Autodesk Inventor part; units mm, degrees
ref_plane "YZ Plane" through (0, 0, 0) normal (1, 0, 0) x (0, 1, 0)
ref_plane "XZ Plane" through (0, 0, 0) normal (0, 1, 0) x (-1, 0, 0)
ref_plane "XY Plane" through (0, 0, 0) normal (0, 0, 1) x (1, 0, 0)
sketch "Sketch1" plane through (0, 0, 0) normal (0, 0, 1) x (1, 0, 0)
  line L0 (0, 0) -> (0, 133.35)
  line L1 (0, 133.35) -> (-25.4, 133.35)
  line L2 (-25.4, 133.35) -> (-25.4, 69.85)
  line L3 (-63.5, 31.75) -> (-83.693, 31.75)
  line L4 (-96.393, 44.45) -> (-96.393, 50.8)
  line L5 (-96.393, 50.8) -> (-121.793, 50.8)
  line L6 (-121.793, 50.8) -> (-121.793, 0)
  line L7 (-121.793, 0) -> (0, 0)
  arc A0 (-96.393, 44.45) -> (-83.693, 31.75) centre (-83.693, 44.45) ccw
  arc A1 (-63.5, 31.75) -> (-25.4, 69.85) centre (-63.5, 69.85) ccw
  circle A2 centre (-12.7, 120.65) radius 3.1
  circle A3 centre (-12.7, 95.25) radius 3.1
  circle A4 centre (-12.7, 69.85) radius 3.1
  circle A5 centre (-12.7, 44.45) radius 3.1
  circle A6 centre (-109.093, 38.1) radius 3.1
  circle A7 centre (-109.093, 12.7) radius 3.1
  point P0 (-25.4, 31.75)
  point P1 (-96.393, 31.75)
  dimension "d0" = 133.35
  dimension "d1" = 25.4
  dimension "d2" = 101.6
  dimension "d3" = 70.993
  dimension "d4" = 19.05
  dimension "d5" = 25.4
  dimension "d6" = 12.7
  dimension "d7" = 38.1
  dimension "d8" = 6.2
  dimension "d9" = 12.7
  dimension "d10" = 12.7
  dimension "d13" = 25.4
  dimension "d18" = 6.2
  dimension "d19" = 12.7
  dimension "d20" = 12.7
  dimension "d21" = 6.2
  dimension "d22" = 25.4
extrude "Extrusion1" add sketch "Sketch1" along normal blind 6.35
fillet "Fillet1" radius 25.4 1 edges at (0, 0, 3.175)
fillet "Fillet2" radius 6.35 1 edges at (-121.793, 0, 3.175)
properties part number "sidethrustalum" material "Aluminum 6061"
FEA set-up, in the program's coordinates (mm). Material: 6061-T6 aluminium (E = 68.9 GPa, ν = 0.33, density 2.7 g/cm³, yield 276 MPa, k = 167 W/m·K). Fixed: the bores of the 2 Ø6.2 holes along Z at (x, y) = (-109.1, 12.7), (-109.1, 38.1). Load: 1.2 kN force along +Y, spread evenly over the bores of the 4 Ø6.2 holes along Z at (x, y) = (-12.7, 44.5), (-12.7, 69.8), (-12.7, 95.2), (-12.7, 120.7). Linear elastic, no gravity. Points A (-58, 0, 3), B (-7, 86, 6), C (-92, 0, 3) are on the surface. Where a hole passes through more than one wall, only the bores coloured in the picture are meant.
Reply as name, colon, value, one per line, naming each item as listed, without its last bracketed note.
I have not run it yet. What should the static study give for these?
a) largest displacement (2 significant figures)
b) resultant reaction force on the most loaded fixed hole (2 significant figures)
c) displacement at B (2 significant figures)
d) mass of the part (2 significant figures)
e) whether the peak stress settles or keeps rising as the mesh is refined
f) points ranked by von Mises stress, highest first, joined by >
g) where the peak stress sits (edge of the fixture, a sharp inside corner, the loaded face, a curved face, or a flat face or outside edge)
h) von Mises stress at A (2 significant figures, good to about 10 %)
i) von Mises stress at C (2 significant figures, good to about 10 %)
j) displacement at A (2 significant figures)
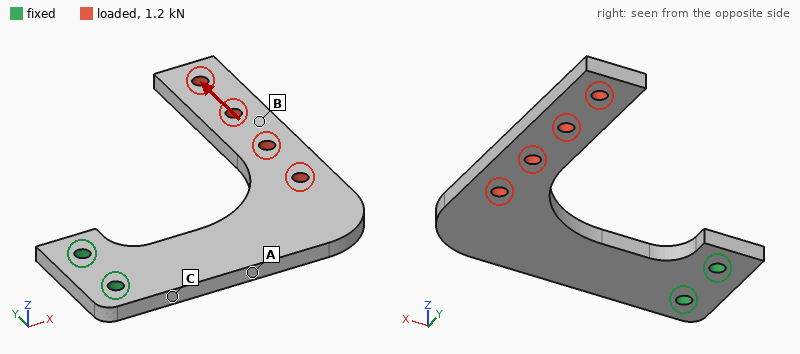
largest displacement: 0.59 mm
resultant reaction force on the most loaded fixed hole: 4.3 kN
displacement at B: 0.42 mm
mass of the part: 120 g
whether the peak stress settles or keeps rising as the mesh is refined: keeps rising
points ranked by von Mises stress, highest first, joined by >: C > A > B
where the peak stress sits: edge of the fixture
von Mises stress at A: 49 MPa
von Mises stress at C: 70 MPa
displacement at A: 0.11 mm
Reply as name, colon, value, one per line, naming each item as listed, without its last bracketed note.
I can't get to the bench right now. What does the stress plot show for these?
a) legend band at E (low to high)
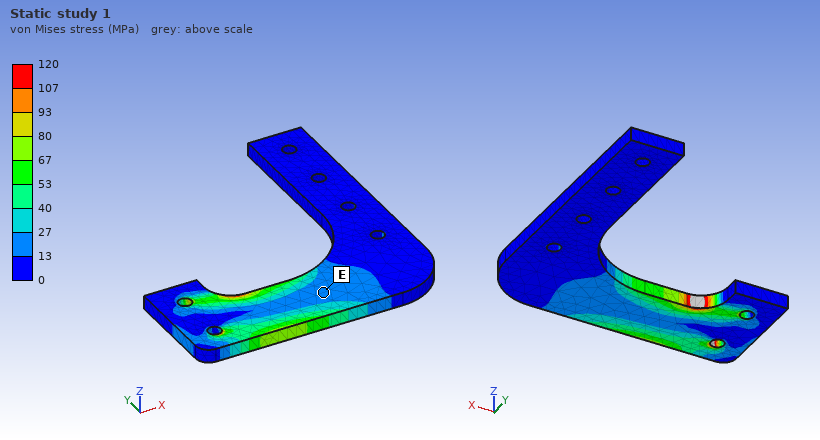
legend band at E: 13 to 27 MPa
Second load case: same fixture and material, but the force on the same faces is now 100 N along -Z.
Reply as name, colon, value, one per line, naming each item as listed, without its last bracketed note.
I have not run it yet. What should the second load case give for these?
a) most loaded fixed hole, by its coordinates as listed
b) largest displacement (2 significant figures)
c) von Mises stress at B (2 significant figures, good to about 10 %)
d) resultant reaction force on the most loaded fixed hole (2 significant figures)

most loaded fixed hole, by its coordinates as listed: (-109.1, 38.1)
largest displacement: 1.9 mm
von Mises stress at B: 6.8 MPa
resultant reaction force on the most loaded fixed hole: 220 N
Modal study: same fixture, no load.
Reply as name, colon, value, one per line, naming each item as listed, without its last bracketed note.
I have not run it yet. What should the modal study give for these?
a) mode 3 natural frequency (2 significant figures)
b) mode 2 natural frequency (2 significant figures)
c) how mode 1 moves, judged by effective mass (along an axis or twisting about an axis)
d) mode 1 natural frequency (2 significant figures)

mode 3 natural frequency: 930 Hz
mode 2 natural frequency: 510 Hz
how mode 1 moves, judged by effective mass: along Z
mode 1 natural frequency: 210 Hz
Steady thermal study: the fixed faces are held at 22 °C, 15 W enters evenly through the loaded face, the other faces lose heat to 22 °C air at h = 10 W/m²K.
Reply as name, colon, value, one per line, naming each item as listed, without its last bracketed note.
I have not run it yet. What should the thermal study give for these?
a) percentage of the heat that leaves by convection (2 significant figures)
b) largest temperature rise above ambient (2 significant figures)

percentage of the heat that leaves by convection: 27 %
largest temperature rise above ambient: 50 K
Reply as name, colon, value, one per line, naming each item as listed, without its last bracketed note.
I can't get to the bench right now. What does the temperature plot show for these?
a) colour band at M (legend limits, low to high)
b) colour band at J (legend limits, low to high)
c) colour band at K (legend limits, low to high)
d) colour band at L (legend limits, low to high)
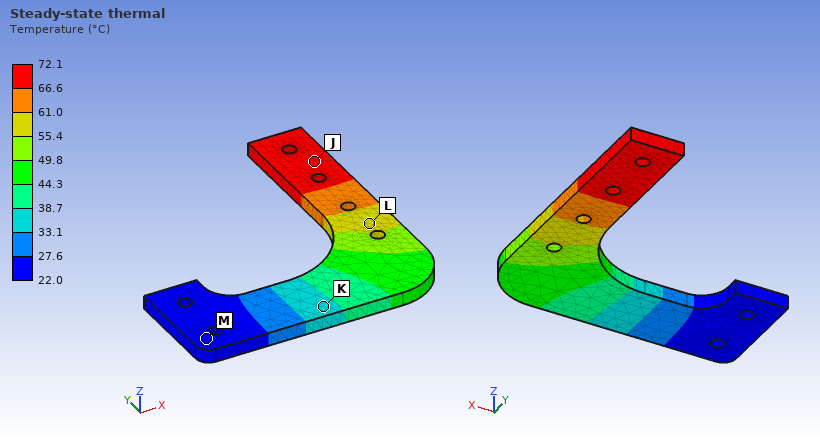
colour band at M: 22.0 to 27.6 °C
colour band at J: 66.6 to 72.1 °C
colour band at K: 33.1 to 38.7 °C
colour band at L: 55.4 to 61.0 °C
